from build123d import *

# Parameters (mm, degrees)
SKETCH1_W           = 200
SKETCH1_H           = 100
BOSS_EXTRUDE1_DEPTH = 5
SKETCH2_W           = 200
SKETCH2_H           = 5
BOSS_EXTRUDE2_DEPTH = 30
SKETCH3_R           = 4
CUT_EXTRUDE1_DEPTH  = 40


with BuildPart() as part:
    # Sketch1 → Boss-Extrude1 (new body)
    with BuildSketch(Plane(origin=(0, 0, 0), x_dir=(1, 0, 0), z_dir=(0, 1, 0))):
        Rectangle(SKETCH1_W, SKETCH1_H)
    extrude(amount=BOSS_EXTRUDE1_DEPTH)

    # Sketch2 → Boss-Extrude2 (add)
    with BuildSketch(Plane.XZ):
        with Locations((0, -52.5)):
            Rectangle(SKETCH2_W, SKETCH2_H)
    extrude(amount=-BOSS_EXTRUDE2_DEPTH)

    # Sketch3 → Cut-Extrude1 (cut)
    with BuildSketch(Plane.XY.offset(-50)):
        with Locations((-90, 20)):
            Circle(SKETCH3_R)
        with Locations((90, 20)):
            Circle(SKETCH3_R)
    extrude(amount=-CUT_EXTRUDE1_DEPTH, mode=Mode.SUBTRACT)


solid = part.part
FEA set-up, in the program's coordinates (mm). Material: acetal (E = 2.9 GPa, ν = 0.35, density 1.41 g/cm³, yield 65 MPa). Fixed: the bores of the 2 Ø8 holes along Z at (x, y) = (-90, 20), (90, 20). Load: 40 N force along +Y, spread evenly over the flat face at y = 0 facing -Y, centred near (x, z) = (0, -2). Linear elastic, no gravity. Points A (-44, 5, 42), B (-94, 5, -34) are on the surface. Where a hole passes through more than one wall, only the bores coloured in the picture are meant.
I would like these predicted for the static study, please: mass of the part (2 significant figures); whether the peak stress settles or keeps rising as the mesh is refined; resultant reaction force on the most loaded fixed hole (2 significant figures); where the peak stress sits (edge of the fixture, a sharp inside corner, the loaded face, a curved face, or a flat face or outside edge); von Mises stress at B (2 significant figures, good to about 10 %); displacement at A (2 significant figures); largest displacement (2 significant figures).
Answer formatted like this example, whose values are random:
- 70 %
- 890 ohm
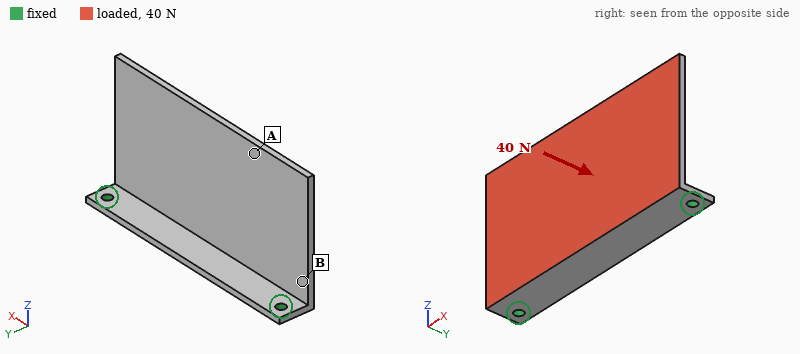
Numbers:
- 180 g
- keeps rising
- 25 N
- edge of the fixture
- 2.2 MPa
- 2.2 mm
- 2.5 mm
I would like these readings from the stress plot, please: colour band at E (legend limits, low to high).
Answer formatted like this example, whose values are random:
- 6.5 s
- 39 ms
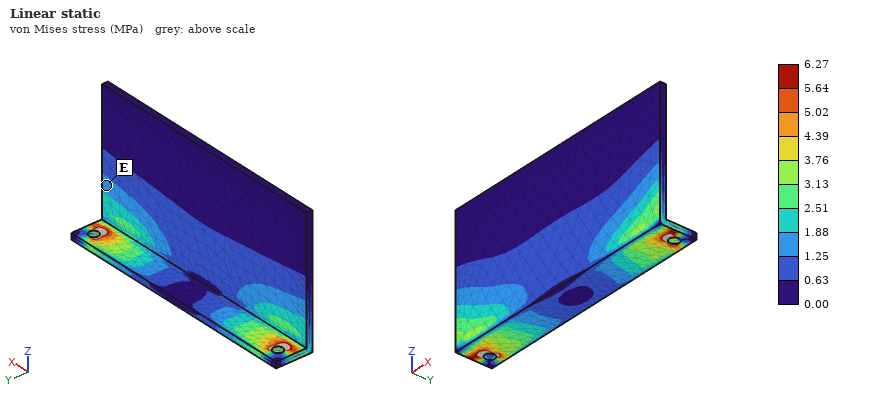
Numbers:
- 1.25 to 1.88 MPa
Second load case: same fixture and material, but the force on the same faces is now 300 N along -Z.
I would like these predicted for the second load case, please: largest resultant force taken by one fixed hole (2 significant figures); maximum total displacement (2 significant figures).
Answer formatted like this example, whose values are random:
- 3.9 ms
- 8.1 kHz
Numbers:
- 150 N
- 2.7 mm
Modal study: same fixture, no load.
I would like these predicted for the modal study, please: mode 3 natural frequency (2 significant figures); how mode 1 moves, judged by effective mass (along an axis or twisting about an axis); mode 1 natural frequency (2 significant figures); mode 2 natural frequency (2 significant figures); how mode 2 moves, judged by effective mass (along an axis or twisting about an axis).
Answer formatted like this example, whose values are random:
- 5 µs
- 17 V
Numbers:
- 310 Hz
- along Y
- 66 Hz
- 150 Hz
- twisting about Z
